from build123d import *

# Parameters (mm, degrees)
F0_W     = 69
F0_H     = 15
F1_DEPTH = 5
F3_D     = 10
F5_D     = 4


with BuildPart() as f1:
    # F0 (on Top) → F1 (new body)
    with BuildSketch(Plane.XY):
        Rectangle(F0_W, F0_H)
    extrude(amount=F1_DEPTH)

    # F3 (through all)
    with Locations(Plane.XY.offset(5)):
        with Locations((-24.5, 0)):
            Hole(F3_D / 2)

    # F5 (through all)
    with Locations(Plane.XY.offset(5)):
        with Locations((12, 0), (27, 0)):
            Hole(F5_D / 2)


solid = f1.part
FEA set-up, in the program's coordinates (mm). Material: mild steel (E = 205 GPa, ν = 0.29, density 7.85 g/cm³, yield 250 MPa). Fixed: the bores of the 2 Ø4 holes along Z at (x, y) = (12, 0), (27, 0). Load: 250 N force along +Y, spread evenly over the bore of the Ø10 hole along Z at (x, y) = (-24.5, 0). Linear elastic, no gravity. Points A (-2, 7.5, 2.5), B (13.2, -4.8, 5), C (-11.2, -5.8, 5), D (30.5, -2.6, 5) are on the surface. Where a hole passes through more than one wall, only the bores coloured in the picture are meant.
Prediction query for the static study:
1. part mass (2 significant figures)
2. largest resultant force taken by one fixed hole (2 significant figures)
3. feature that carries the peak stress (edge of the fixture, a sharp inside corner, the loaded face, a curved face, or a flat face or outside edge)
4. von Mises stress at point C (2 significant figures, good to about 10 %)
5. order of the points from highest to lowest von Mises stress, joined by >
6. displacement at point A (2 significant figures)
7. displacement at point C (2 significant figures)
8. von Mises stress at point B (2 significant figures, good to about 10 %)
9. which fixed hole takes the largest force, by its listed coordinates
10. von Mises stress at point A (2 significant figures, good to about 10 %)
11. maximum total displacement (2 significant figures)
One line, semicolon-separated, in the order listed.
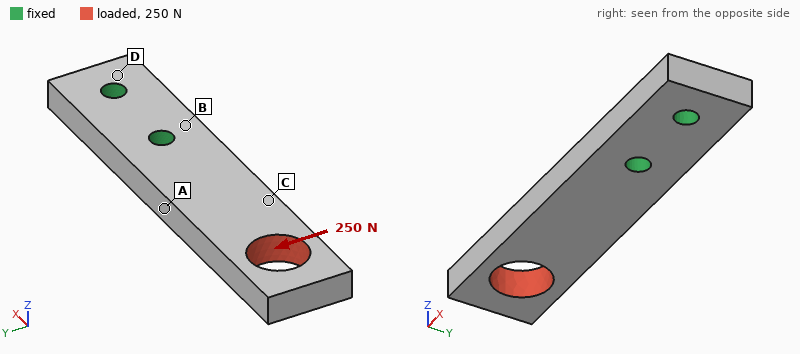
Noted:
37 g; 600 N; edge of the fixture; 14 MPa; A > B > C > D; 6.9 µm; 12 µm; 24 MPa; (12, 0); 30 MPa; 32 µm
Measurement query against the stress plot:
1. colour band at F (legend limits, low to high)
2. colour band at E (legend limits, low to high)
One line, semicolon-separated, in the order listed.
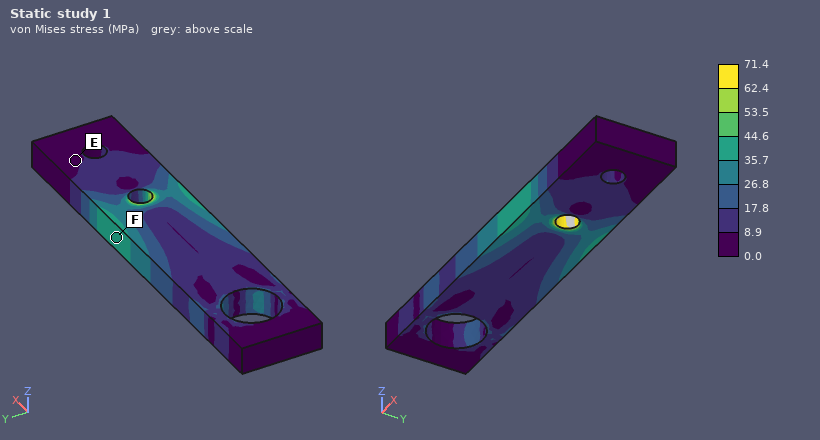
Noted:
35.7 to 44.6 MPa; 0.0 to 8.9 MPa
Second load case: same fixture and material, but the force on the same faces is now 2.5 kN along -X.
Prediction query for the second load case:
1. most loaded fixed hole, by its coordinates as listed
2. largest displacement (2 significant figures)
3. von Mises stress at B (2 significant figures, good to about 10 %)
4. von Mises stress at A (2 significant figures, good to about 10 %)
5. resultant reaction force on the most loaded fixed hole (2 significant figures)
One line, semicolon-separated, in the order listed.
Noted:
(12, 0); 10 µm; 17 MPa; 33 MPa; 2.2 kN
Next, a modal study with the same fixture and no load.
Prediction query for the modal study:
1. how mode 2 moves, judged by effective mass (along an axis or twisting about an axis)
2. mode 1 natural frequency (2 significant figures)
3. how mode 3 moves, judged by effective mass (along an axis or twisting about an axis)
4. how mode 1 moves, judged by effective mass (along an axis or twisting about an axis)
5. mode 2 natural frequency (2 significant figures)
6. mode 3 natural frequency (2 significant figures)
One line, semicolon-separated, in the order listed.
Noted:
along Y; 2200 Hz; twisting about X; along Z; 5000 Hz; 9700 Hz
